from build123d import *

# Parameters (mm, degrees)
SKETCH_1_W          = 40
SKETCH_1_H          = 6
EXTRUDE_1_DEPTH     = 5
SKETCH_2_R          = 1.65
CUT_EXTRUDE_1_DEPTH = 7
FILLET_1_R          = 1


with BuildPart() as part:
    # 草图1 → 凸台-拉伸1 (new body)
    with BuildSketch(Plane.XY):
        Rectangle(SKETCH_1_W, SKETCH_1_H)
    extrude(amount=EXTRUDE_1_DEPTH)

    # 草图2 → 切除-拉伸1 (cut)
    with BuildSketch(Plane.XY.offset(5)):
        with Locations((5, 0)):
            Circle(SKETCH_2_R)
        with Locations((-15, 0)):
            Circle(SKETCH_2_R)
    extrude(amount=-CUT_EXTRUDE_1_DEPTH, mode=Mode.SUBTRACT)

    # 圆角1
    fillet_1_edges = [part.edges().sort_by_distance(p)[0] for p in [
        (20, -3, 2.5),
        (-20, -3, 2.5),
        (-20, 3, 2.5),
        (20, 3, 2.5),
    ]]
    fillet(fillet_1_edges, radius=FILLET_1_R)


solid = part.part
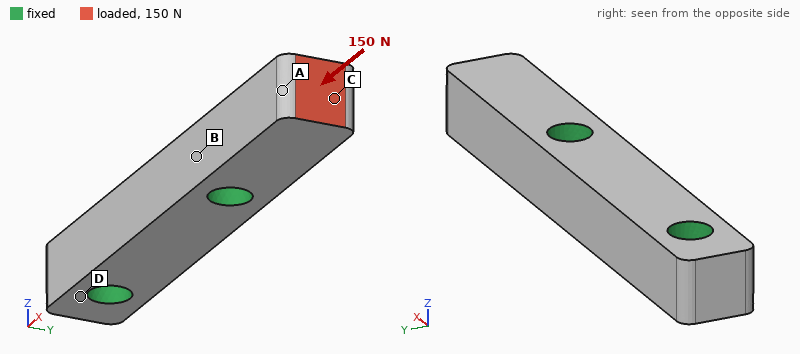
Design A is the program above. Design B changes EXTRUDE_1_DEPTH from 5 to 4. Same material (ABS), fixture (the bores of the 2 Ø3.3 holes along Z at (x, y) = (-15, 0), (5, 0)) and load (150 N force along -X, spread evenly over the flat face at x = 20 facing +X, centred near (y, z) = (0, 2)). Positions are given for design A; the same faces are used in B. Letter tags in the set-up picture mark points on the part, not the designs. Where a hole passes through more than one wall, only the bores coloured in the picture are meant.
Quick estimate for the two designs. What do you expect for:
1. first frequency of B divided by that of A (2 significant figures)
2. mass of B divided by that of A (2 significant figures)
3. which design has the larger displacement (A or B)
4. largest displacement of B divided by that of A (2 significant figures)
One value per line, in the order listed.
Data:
0.83
0.80
B
1.2
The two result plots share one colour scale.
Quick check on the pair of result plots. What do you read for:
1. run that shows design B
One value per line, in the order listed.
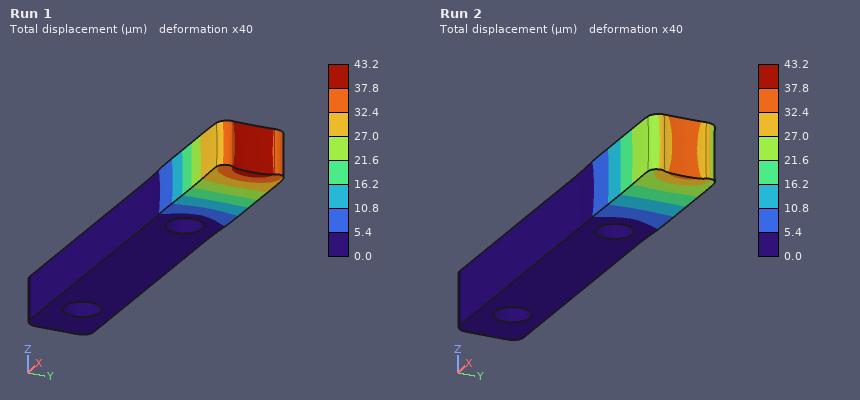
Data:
Run 1
